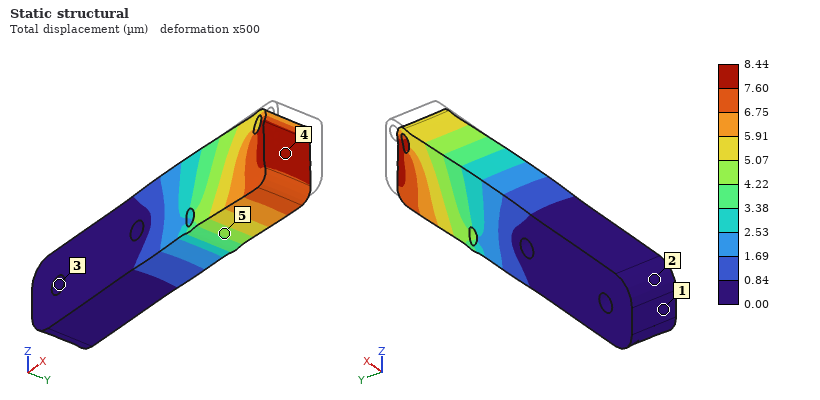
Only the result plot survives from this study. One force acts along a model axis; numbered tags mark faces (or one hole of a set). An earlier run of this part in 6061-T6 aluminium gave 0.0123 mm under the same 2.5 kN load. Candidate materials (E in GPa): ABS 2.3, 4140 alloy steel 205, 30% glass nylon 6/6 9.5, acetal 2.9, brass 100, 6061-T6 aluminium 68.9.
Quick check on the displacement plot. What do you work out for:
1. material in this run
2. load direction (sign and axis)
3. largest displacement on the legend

brass
-X
8.44 µm
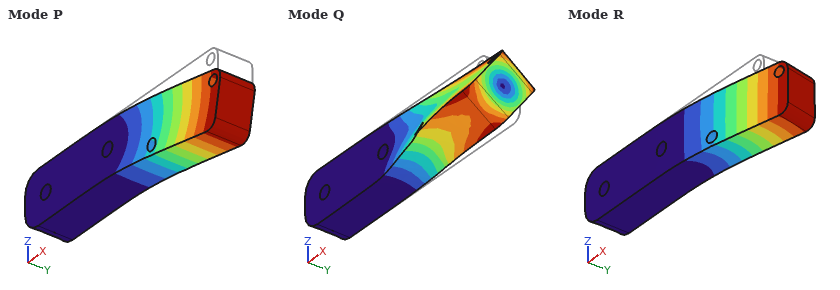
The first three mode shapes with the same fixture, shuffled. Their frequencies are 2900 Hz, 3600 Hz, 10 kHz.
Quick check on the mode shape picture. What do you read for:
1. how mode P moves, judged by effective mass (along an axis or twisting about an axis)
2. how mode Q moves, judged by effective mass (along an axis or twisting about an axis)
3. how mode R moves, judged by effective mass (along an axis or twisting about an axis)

along Z
twisting about X
along Y
